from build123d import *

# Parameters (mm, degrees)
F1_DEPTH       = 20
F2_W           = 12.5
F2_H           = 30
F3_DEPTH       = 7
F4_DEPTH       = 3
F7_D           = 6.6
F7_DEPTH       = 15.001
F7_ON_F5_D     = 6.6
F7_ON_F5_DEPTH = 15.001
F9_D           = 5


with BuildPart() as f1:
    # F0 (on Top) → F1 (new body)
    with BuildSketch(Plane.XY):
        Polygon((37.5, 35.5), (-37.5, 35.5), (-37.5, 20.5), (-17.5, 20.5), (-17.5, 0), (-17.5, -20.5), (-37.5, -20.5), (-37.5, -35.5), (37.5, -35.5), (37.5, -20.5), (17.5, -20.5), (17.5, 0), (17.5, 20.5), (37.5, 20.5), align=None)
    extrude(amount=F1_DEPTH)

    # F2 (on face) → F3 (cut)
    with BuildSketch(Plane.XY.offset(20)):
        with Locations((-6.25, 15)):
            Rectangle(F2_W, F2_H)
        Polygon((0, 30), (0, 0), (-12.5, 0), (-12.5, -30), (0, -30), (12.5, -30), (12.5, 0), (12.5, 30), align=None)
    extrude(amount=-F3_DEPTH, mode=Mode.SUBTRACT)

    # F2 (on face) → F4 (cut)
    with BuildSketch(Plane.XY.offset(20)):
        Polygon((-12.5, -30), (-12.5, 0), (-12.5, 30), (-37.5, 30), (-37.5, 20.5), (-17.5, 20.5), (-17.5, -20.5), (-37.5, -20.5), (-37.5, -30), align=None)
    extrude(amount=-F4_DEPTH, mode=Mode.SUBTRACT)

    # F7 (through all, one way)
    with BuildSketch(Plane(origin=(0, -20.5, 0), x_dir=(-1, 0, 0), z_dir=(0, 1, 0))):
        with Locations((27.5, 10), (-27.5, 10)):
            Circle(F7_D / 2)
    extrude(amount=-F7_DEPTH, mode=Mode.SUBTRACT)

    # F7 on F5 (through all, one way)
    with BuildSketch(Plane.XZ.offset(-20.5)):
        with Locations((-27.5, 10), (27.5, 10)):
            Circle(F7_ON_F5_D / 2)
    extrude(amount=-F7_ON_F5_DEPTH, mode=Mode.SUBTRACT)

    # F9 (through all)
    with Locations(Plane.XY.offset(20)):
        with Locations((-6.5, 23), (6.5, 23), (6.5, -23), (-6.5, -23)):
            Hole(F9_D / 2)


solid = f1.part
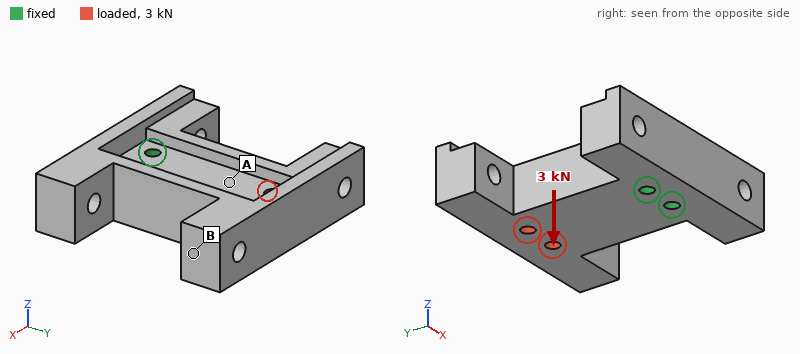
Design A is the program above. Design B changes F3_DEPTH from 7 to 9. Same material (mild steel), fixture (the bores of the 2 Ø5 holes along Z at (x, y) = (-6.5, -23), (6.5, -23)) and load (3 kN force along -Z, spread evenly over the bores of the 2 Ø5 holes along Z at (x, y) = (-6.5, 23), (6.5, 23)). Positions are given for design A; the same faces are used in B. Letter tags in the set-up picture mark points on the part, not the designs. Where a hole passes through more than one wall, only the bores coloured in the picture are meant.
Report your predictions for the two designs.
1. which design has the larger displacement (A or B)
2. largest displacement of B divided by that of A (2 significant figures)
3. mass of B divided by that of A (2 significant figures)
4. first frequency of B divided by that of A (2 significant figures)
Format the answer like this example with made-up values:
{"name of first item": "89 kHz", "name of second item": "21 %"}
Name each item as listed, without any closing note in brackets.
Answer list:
{"which design has the larger displacement": "B", "largest displacement of B divided by that of A": "1.3", "mass of B divided by that of A": "0.95", "first frequency of B divided by that of A": "0.89"}
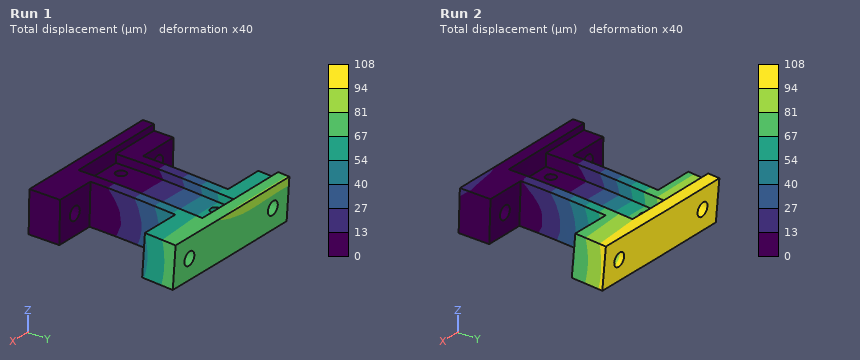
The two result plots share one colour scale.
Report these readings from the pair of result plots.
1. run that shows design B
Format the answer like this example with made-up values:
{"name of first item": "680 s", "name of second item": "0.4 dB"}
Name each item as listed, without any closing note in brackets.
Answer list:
{"run that shows design B": "Run 2"}
